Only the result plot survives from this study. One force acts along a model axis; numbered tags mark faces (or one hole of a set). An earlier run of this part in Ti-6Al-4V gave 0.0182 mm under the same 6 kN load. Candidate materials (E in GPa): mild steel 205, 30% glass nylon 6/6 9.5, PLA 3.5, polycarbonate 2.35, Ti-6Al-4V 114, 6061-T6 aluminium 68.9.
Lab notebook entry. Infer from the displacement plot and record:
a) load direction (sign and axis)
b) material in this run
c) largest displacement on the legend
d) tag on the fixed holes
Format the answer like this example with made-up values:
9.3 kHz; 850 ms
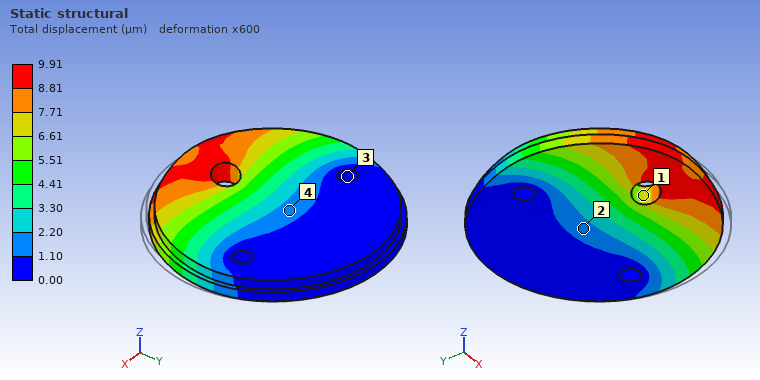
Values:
-X; mild steel; 9.91 µm; 3
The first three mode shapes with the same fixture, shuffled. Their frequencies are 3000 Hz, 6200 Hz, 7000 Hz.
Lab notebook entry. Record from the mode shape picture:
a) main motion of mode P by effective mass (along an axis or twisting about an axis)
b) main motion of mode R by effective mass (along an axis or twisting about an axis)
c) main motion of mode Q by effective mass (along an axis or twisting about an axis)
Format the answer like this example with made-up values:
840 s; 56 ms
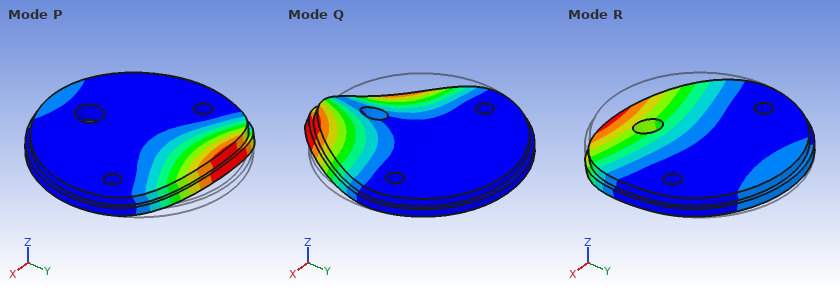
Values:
along Z; along Z; twisting about Y
